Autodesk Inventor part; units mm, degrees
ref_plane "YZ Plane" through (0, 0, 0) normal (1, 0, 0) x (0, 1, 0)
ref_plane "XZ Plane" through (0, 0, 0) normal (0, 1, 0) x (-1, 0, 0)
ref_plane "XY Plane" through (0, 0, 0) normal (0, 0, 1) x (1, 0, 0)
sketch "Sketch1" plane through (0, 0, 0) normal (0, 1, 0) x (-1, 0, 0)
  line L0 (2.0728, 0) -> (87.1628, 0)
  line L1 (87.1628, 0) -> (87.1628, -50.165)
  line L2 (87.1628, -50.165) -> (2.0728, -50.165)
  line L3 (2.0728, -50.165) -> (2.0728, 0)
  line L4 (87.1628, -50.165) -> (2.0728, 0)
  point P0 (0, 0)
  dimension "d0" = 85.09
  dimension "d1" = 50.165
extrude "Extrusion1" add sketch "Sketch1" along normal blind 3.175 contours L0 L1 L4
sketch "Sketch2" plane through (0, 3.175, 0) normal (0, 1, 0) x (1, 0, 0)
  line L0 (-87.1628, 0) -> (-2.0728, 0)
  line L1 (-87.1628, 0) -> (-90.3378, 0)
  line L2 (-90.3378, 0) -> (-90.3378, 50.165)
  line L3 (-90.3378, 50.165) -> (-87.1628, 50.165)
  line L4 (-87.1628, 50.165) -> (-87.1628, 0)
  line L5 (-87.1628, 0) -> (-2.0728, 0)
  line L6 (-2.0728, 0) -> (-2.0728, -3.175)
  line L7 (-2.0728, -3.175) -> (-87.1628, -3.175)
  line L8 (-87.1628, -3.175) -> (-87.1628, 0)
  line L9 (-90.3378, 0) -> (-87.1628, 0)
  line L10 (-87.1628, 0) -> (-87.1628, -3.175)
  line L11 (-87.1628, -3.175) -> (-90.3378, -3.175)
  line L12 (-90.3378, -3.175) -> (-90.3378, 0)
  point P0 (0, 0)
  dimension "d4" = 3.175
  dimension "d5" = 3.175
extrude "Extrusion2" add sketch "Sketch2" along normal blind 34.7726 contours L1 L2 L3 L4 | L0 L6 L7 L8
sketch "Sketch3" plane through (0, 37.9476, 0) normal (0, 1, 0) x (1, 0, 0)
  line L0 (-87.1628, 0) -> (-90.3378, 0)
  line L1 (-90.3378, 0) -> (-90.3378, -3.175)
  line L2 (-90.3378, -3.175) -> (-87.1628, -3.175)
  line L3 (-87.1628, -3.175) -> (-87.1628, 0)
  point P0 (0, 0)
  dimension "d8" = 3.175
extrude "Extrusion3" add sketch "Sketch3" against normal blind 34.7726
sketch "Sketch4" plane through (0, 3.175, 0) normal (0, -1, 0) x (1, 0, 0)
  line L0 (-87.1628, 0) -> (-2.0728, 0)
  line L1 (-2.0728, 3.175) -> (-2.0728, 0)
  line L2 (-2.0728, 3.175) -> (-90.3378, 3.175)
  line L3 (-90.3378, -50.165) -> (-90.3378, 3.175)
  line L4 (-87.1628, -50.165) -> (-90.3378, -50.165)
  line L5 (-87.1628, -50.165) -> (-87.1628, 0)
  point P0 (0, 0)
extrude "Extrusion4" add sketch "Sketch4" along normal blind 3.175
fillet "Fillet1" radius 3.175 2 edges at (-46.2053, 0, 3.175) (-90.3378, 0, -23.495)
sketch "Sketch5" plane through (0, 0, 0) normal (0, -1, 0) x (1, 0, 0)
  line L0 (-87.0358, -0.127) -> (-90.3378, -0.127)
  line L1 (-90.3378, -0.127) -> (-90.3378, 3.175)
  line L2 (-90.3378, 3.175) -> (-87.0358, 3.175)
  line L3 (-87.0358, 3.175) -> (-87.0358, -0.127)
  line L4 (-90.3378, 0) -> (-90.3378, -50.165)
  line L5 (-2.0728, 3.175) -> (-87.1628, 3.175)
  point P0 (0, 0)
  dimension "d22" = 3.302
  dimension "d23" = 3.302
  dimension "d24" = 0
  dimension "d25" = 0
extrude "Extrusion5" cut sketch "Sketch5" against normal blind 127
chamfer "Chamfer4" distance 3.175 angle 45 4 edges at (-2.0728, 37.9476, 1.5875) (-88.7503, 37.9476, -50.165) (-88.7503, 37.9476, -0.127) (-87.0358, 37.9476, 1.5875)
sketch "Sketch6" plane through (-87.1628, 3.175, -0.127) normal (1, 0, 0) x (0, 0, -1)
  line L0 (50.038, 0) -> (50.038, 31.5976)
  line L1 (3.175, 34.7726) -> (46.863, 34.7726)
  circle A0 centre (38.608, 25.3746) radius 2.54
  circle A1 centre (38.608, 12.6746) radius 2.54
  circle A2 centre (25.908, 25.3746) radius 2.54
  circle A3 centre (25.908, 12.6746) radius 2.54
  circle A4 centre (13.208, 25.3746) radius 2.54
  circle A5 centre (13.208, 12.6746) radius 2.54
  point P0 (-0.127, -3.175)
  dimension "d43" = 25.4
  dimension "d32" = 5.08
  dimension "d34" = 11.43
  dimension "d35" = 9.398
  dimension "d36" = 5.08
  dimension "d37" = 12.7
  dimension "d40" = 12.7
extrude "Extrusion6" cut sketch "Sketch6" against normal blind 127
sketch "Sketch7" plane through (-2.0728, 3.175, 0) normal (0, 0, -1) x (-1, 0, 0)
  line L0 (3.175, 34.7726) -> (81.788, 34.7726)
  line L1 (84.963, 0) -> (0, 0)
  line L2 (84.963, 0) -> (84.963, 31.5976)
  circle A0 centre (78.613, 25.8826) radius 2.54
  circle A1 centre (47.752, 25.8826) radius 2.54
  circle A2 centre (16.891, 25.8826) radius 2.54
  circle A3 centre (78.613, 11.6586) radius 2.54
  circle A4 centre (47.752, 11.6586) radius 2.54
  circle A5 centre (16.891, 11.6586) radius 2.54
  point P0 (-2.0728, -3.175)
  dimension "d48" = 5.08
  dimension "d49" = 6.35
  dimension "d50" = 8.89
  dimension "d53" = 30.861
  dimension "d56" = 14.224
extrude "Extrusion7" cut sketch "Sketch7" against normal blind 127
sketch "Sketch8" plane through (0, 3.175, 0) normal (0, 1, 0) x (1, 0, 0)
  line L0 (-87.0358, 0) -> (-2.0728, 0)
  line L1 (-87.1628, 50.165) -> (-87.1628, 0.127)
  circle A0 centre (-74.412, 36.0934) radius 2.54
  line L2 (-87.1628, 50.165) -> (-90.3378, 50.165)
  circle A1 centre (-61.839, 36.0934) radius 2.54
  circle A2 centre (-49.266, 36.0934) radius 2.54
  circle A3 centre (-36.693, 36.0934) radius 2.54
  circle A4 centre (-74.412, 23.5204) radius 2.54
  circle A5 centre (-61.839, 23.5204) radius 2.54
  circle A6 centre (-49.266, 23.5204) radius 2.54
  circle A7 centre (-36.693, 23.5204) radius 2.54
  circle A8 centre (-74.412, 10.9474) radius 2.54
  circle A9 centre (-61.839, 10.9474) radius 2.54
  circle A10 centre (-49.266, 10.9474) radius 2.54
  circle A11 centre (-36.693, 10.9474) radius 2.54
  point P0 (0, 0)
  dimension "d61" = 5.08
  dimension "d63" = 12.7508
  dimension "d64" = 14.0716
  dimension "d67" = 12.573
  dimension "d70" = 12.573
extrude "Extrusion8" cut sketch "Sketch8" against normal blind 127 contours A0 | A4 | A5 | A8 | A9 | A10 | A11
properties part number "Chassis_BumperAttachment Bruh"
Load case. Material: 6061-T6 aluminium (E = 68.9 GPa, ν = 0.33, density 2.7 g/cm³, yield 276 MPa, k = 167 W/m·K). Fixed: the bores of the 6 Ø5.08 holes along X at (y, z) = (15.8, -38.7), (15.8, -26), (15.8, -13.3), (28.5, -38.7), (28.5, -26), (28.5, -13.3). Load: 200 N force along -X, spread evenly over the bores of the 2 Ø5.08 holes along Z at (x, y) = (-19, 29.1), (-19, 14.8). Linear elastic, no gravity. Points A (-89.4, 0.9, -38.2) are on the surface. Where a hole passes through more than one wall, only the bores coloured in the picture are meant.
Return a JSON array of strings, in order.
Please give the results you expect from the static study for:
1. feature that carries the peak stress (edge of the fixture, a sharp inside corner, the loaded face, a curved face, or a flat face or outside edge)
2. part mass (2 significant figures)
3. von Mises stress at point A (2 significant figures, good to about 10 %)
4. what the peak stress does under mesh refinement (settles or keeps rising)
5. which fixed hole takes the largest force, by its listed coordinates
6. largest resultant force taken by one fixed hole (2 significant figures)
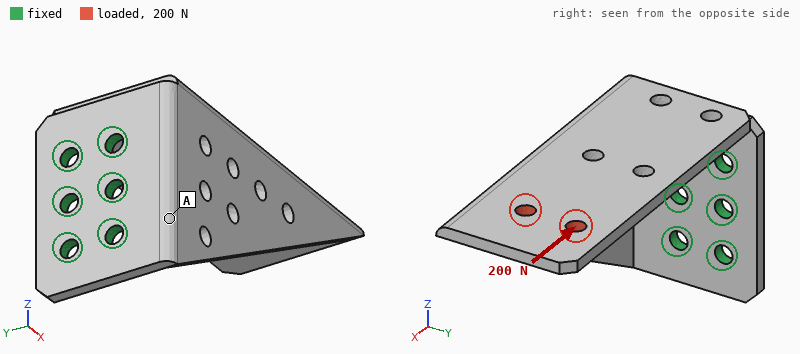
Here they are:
["a sharp inside corner", "58 g", "7.7 MPa", "keeps rising", "(15.8, -13.3)", "260 N"]
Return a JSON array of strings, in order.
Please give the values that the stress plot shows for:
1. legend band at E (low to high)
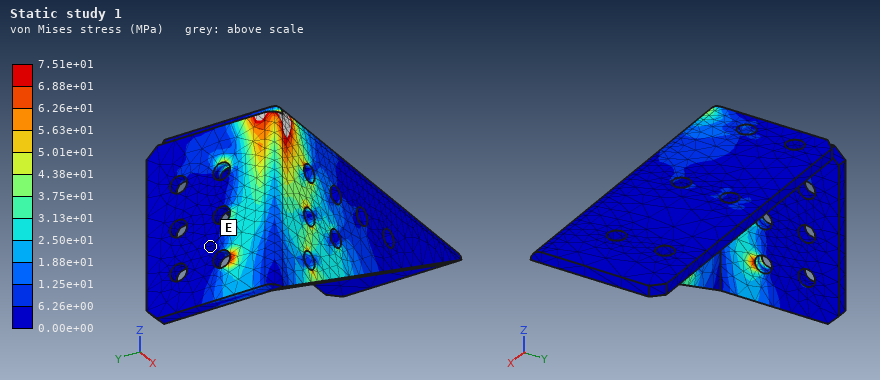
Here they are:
["0.00e+00 to 6.26e+00 MPa"]
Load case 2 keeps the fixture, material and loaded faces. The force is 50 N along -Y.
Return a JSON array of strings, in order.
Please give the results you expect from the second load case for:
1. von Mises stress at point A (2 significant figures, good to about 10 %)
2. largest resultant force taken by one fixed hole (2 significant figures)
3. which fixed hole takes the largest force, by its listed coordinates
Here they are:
["16 MPa", "60 N", "(15.8, -13.3)"]
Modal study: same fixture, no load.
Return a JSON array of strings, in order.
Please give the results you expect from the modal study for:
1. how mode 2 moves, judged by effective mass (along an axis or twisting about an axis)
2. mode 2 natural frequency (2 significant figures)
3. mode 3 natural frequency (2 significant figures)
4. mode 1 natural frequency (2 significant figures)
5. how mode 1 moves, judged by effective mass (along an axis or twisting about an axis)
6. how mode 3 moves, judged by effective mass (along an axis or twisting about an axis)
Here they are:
["along Z", "670 Hz", "1400 Hz", "280 Hz", "along Y", "along X"]
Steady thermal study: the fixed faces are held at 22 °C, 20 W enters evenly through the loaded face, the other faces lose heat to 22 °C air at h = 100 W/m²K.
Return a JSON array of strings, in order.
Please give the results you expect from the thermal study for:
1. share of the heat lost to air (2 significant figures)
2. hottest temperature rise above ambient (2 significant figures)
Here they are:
["80 %", "33 K"]
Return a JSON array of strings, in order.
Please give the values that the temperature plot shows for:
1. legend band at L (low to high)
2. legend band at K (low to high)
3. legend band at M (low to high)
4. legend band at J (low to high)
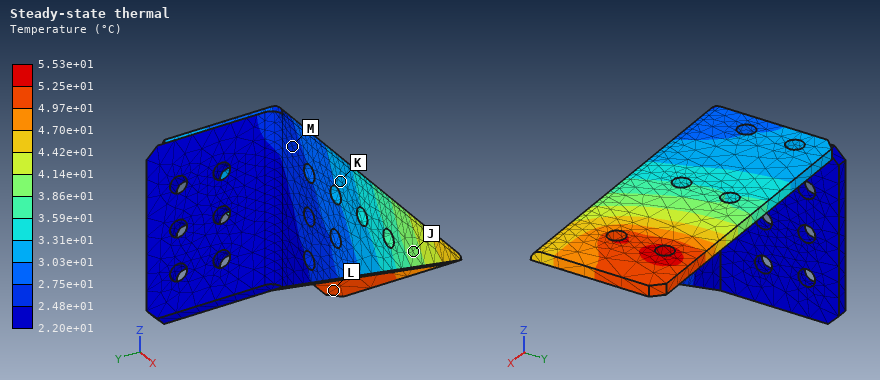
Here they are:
["4.97e+01 to 5.25e+01 °C", "3.03e+01 to 3.31e+01 °C", "2.48e+01 to 2.75e+01 °C", "3.86e+01 to 4.14e+01 °C"]
